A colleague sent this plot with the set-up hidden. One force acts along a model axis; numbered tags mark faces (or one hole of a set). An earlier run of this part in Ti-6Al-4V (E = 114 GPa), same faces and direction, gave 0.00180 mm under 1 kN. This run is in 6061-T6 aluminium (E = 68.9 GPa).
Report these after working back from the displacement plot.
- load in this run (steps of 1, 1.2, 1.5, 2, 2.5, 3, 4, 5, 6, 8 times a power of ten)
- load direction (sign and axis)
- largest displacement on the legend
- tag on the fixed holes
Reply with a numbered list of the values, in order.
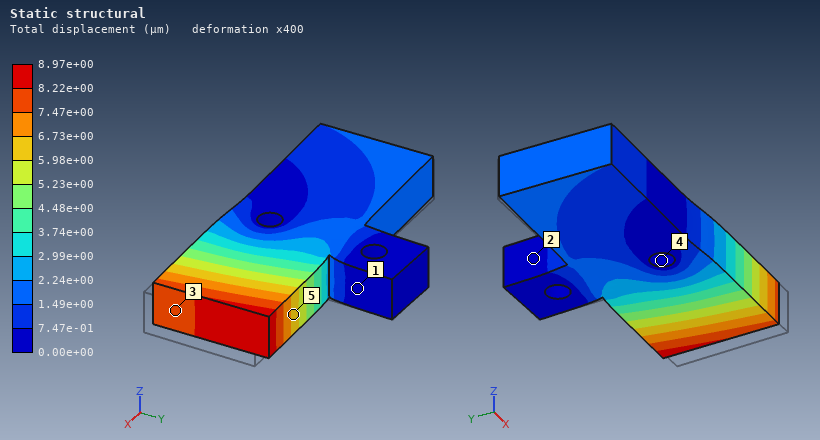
1. 3 kN
2. -X
3. 8.97e+00 µm
4. 4
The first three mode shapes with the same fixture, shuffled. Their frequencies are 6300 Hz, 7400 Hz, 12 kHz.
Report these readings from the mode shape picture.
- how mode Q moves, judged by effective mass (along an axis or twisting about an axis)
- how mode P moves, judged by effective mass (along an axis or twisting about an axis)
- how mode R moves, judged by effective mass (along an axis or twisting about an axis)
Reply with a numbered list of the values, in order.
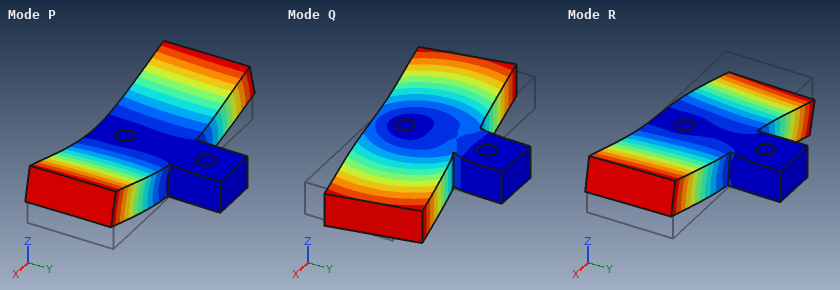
1. twisting about Z
2. along Z
3. twisting about Y
